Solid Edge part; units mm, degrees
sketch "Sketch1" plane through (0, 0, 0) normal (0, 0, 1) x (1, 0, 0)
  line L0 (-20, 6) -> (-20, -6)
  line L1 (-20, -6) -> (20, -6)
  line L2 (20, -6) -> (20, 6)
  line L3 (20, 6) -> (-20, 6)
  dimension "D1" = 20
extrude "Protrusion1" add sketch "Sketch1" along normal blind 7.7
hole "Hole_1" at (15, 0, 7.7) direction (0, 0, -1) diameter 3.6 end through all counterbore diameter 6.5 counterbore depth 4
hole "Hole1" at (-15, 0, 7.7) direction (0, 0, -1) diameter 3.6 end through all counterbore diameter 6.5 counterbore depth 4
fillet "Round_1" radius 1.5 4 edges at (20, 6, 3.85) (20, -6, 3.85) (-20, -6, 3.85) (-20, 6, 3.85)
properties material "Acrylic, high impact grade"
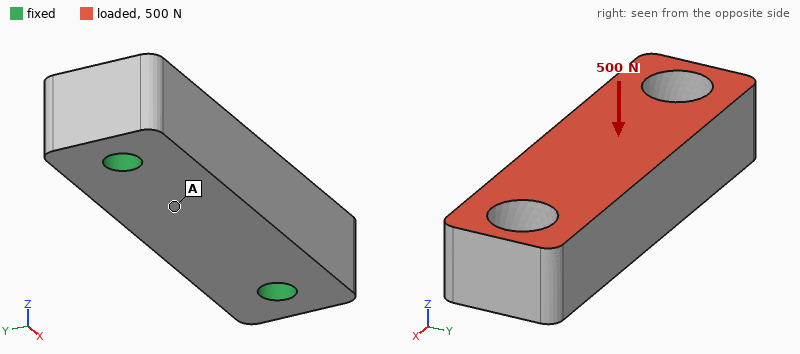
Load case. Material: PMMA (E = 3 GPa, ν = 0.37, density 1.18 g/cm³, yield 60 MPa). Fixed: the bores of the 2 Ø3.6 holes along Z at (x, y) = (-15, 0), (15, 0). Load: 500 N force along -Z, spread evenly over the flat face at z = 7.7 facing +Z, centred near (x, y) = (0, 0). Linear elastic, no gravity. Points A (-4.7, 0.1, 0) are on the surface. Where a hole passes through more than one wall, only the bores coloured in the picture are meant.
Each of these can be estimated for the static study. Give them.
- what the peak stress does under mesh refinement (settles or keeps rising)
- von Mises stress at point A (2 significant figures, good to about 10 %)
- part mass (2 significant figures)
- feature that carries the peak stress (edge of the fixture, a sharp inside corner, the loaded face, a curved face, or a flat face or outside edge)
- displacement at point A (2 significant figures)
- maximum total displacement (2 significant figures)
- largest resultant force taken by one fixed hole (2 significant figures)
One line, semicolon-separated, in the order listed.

keeps rising; 4.0 MPa; 3.9 g; edge of the fixture; 53 µm; 64 µm; 270 N
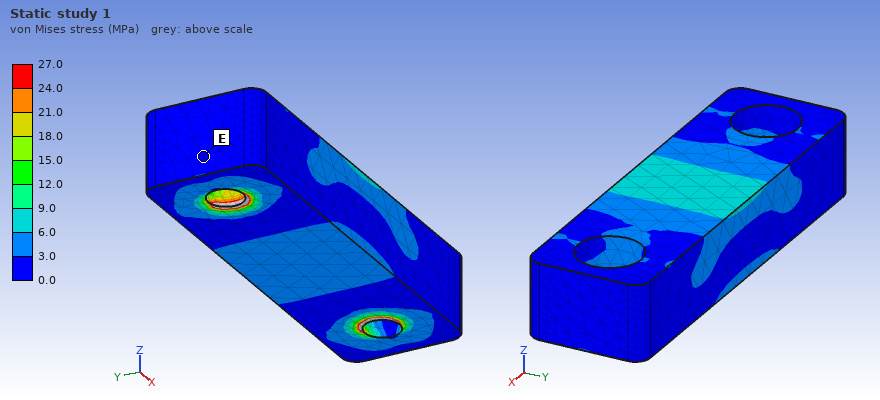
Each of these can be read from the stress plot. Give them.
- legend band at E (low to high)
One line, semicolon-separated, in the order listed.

0.0 to 3.0 MPa
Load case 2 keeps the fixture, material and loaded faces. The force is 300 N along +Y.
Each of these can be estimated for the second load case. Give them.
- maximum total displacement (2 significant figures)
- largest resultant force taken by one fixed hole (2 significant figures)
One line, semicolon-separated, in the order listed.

0.10 mm; 150 N
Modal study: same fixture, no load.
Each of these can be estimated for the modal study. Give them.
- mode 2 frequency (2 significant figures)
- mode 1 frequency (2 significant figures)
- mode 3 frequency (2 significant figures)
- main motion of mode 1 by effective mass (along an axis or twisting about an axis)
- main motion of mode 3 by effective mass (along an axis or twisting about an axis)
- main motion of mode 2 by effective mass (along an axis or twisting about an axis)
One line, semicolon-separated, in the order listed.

8000 Hz; 7500 Hz; 10 kHz; along Y; along Y; along Z
